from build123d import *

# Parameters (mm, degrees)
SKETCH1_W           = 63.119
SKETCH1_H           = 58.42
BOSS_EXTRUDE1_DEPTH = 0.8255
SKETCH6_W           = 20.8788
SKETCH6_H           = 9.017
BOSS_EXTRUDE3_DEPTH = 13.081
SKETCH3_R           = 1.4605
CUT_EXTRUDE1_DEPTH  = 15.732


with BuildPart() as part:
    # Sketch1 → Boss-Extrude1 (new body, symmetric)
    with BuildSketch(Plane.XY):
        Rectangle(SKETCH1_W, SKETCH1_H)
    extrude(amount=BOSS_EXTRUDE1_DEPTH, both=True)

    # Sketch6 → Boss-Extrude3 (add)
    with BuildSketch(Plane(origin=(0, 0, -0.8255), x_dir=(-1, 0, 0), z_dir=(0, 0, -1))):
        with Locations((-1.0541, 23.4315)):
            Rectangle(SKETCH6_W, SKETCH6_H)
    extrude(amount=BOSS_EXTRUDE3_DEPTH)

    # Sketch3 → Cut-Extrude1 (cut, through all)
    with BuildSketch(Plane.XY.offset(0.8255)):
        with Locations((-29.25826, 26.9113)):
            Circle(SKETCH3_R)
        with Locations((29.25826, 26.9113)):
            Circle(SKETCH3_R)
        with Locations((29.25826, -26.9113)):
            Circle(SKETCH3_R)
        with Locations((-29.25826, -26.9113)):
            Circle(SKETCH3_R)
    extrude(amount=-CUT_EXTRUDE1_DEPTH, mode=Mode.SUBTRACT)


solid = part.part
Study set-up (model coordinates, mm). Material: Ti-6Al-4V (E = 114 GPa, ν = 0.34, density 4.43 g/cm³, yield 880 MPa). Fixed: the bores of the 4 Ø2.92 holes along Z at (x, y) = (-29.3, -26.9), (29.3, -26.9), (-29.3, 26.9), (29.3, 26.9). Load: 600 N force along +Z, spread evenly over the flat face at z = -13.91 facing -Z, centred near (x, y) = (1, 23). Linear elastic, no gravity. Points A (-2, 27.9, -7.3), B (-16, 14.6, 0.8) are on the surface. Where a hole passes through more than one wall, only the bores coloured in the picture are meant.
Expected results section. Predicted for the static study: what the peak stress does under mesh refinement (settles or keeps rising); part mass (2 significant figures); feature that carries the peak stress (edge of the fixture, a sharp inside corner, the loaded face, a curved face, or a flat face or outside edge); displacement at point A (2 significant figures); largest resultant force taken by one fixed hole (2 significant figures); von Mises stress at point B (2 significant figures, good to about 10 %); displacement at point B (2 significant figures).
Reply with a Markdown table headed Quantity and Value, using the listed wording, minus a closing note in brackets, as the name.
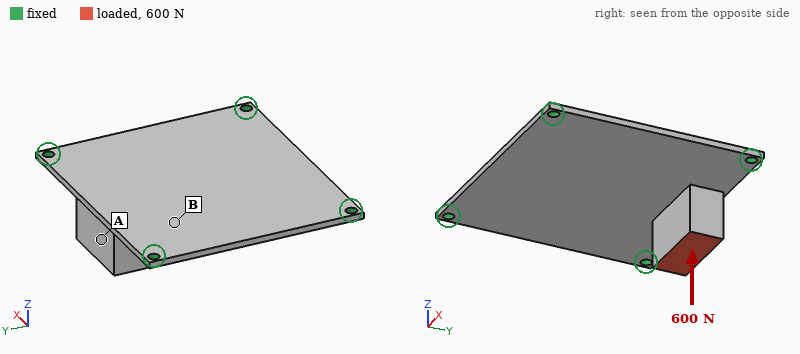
| Quantity | Value |
|---|---|
| what the peak stress does under mesh refinement | keeps rising |
| part mass | 38 g |
| feature that carries the peak stress | edge of the fixture |
| displacement at point A | 0.33 mm |
| largest resultant force taken by one fixed hole | 330 N |
| von Mises stress at point B | 120 MPa |
| displacement at point B | 0.19 mm |
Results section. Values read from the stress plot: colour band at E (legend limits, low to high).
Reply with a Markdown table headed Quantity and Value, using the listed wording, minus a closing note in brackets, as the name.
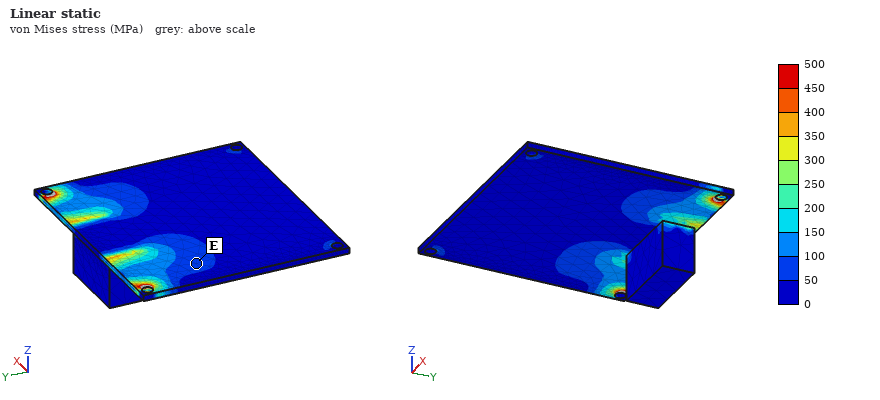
| Quantity | Value |
|---|---|
| colour band at E | 50 to 100 MPa |
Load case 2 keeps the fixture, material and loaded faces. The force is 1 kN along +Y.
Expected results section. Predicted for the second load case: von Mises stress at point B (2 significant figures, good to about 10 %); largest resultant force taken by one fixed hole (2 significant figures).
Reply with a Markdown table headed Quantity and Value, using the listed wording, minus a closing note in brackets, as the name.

| Quantity | Value |
|---|---|
| von Mises stress at point B | 230 MPa |
| largest resultant force taken by one fixed hole | 380 N |
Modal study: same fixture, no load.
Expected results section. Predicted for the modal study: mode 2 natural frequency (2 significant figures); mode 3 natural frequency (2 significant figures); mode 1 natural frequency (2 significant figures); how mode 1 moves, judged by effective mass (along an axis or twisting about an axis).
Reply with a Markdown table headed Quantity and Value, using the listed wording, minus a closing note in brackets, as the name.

| Quantity | Value |
|---|---|
| mode 2 natural frequency | 2000 Hz |
| mode 3 natural frequency | 3000 Hz |
| mode 1 natural frequency | 1600 Hz |
| how mode 1 moves, judged by effective mass | along Z |
